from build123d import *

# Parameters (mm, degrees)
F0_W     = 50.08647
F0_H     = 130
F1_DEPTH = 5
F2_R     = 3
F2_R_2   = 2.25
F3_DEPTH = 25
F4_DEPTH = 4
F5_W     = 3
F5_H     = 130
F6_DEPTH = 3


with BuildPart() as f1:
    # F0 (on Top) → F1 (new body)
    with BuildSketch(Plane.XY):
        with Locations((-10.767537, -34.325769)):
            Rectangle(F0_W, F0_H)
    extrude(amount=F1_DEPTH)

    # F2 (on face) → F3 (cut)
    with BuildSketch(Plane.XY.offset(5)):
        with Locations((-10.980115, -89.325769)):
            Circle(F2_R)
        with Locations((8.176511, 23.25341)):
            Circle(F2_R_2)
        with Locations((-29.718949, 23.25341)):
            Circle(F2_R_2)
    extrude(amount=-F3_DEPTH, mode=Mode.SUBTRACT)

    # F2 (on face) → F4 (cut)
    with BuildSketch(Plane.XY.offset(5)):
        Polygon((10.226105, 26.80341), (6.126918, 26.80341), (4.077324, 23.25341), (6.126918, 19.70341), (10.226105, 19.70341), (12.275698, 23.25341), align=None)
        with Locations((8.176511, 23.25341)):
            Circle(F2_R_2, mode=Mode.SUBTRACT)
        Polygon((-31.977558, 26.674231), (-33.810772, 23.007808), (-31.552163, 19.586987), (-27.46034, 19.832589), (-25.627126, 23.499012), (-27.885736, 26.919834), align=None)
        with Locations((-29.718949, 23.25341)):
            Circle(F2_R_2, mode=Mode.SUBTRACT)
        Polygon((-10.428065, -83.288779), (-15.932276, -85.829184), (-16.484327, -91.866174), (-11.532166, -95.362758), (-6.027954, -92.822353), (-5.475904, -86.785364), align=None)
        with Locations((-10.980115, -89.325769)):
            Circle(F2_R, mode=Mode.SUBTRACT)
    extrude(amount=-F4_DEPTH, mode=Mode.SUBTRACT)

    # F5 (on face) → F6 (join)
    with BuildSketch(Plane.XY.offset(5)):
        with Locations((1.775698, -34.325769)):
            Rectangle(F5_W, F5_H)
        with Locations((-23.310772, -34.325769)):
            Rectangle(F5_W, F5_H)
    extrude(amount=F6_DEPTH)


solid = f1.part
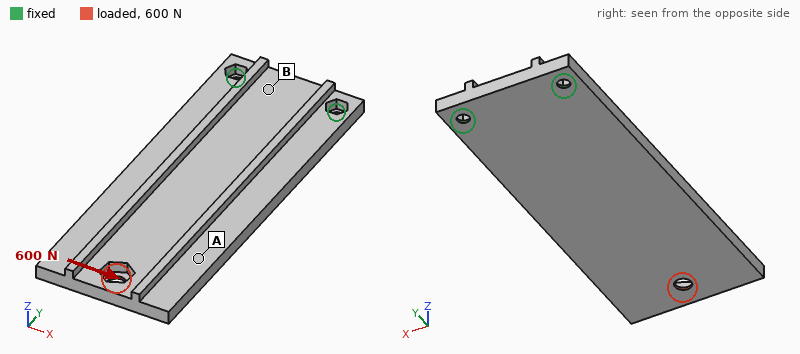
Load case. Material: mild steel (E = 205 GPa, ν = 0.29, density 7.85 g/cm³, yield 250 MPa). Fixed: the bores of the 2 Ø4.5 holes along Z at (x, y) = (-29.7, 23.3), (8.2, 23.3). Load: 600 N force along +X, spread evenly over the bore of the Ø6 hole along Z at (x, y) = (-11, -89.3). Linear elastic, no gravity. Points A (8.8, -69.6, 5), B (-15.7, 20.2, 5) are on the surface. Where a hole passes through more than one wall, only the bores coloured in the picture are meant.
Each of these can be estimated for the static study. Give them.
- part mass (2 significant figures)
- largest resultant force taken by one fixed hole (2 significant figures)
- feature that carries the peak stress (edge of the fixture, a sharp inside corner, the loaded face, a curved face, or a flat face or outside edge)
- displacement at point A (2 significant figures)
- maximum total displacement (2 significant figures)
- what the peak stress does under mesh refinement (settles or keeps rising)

270 g
1.7 kN
edge of the fixture
43 µm
68 µm
keeps rising
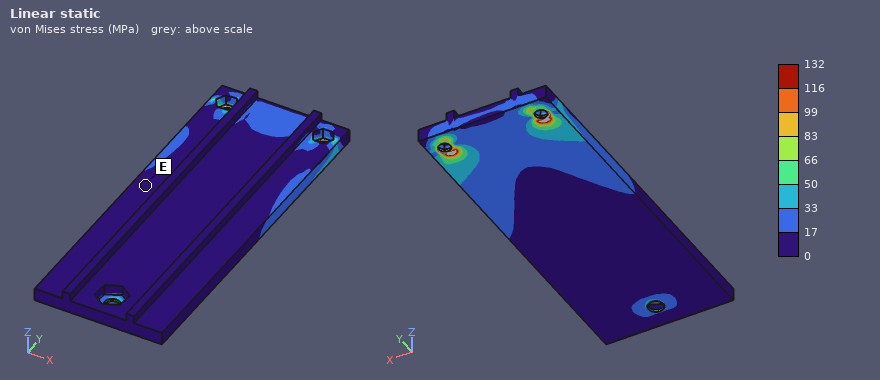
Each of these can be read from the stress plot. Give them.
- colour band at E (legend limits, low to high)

0 to 17 MPa
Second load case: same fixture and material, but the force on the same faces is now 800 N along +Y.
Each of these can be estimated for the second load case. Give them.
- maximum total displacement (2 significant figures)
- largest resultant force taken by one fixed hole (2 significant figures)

76 µm
410 N
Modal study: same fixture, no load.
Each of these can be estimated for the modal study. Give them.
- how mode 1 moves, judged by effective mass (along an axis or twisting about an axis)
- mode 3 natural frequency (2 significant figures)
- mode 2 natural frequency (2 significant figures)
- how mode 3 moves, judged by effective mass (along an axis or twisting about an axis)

along Z
1600 Hz
1300 Hz
along Z
